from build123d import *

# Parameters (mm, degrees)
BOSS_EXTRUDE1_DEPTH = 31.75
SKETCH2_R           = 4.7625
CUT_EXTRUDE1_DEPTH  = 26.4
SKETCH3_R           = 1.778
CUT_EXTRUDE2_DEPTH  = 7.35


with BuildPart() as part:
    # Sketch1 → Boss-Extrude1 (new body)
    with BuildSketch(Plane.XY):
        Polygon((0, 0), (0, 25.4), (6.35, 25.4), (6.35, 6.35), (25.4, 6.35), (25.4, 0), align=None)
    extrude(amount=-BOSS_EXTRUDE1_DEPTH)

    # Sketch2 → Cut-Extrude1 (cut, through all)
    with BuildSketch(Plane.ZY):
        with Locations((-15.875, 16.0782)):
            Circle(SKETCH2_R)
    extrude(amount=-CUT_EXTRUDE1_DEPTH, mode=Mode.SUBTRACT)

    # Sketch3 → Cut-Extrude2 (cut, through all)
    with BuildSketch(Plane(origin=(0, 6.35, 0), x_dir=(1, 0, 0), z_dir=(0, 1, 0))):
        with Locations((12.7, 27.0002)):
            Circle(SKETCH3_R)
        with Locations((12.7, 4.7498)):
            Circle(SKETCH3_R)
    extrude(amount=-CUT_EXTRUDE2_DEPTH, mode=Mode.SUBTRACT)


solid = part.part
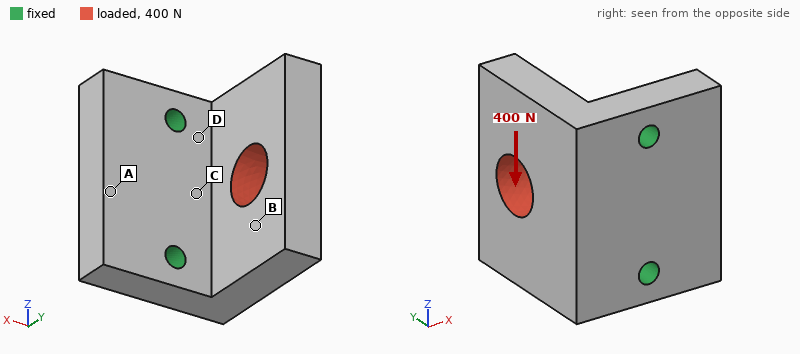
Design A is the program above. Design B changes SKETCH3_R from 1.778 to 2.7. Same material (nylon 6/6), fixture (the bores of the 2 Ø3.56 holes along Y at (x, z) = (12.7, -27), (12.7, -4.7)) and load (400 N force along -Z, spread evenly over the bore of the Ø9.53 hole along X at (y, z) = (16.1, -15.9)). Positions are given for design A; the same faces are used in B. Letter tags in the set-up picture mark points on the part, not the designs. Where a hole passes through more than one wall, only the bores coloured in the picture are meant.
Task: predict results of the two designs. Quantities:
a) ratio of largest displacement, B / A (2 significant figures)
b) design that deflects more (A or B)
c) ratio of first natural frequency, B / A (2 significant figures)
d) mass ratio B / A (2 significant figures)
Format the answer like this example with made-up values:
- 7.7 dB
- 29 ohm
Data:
- 0.84
- A
- 1.1
- 0.98
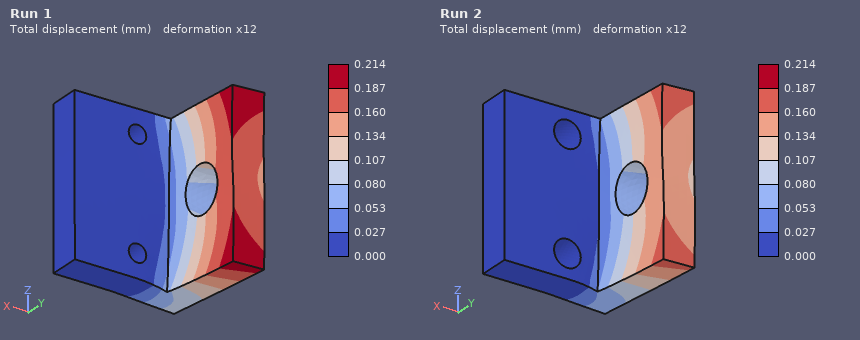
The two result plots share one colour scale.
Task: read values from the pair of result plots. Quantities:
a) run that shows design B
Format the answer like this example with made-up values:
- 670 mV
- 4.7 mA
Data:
- Run 2
